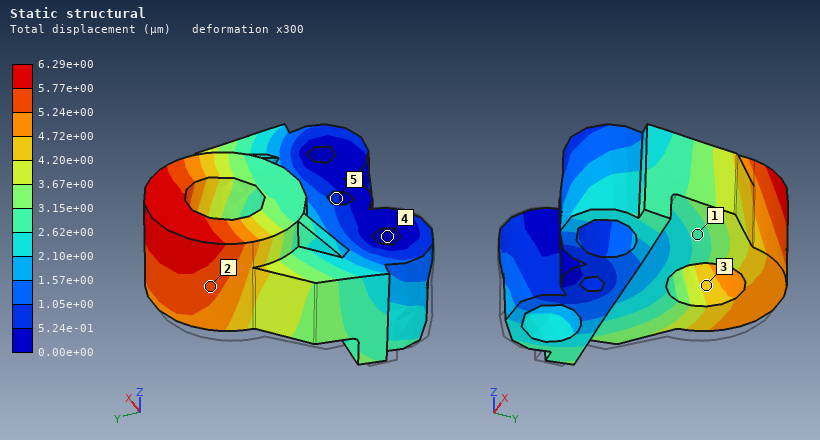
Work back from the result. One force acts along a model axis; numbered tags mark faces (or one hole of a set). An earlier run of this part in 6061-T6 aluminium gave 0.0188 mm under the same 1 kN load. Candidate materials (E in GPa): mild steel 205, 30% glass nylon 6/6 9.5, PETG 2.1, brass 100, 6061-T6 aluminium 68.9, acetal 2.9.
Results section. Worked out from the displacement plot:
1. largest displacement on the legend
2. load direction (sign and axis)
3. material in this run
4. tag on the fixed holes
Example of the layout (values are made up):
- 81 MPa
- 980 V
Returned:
- 6.29e+00 µm
- +X
- mild steel
- 4
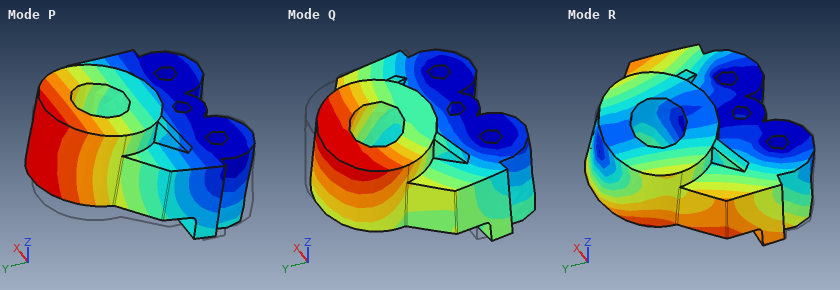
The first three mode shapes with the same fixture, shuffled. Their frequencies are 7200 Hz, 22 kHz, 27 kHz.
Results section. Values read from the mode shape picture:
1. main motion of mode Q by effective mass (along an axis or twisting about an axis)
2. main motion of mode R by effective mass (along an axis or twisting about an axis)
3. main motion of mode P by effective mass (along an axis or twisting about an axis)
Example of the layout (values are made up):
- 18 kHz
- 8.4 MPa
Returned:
- along X
- along X
- along Z
